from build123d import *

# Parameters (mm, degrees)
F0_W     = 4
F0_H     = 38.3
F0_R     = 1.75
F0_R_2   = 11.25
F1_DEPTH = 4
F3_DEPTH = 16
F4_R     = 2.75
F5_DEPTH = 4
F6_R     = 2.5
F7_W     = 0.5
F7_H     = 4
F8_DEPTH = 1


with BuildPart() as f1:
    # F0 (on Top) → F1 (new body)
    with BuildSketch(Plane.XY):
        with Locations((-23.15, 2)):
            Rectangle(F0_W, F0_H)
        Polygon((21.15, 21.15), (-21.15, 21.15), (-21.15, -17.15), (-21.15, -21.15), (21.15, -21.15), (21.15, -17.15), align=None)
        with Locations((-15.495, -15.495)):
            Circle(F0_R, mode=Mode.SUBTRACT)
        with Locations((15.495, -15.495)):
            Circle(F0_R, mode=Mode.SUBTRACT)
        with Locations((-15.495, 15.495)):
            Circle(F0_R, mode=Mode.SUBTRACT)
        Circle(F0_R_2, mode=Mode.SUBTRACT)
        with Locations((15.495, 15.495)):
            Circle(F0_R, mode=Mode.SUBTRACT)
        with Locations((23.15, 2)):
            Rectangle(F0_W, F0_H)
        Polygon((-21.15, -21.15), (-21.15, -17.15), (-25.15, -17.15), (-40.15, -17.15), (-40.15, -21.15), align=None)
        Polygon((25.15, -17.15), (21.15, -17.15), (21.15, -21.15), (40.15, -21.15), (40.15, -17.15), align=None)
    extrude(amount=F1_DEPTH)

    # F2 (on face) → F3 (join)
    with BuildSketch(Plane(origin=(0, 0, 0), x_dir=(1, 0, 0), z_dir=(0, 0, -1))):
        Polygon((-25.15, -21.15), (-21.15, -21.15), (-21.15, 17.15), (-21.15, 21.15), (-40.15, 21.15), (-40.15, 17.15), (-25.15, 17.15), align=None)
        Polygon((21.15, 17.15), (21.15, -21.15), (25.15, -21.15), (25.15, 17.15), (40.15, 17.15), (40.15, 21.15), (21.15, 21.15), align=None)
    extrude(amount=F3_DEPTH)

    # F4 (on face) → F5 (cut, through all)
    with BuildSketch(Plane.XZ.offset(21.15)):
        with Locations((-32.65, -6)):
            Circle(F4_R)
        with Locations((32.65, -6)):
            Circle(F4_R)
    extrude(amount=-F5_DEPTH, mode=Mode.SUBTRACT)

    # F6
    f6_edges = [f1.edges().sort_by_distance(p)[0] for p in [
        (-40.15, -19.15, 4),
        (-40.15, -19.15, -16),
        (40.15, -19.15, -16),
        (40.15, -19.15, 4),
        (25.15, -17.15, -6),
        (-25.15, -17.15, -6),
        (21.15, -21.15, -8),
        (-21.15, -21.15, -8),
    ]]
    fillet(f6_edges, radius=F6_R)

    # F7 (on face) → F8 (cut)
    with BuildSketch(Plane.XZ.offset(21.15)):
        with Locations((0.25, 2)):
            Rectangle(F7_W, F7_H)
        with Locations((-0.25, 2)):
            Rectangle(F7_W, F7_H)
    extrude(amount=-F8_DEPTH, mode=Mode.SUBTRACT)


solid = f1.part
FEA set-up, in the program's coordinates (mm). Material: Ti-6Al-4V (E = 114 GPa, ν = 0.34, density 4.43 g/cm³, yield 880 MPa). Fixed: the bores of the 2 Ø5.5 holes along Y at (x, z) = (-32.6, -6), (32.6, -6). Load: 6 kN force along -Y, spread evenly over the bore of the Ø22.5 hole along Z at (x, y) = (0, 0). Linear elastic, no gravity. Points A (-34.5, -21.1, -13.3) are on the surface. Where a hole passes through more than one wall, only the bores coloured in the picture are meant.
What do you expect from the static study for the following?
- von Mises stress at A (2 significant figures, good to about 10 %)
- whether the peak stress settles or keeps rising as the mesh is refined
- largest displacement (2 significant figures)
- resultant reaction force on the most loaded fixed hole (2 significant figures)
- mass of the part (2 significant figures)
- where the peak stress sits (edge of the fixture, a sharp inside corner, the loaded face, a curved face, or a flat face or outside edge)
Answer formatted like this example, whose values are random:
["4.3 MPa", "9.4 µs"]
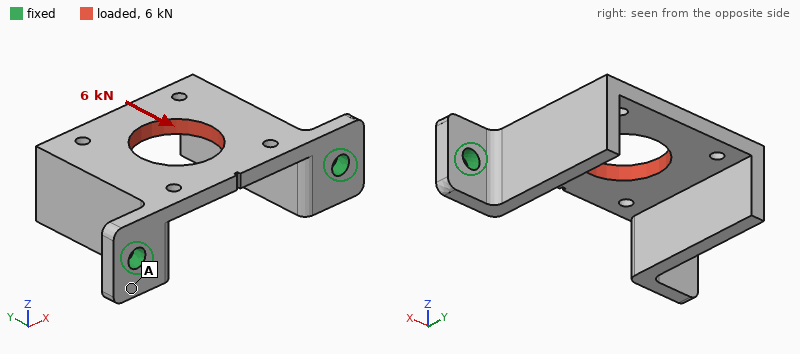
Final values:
["92 MPa", "keeps rising", "0.33 mm", "3.3 kN", "64 g", "edge of the fixture"]
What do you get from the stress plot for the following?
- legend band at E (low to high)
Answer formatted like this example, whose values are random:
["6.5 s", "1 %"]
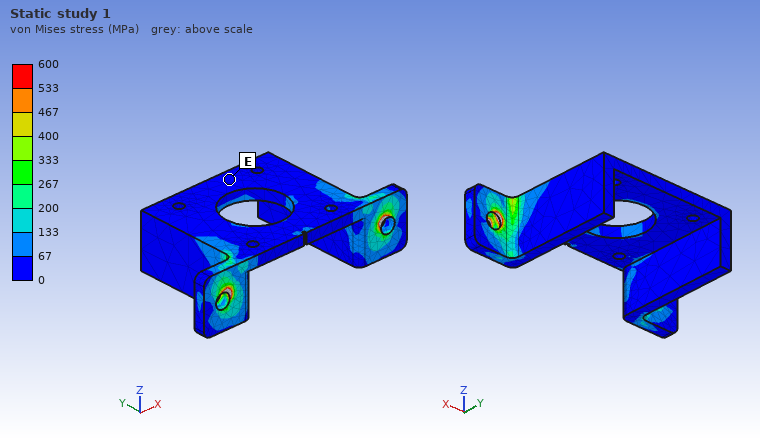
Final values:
["0 to 67 MPa"]
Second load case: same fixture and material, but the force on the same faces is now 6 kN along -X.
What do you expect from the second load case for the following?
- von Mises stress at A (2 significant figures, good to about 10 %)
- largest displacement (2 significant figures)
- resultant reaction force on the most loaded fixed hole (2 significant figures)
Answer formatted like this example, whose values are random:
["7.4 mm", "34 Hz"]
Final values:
["37 MPa", "0.16 mm", "3.6 kN"]
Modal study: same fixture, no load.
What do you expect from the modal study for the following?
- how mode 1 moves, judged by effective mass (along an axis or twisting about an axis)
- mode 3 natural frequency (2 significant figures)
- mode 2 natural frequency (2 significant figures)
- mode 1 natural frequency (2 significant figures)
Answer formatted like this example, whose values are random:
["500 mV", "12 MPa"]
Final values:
["along Z", "5300 Hz", "3000 Hz", "2200 Hz"]
